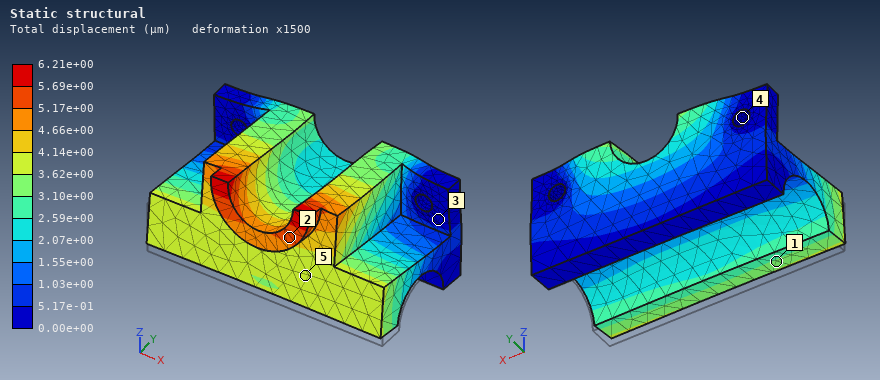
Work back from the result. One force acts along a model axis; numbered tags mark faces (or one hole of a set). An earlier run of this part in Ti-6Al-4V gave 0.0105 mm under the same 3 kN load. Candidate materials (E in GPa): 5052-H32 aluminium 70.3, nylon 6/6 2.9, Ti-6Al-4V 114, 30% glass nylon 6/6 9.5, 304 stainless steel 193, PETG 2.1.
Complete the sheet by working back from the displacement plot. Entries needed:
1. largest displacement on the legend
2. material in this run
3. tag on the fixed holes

6.21e+00 µm
304 stainless steel
4
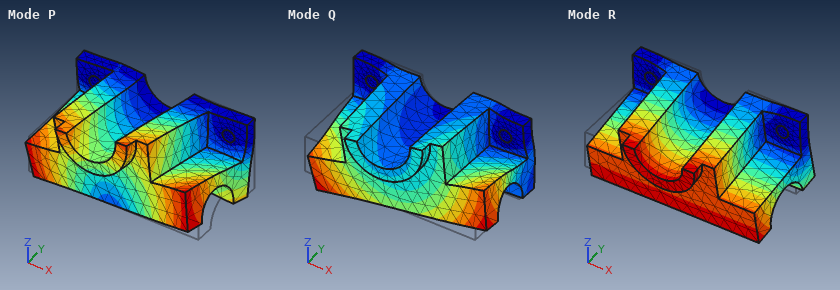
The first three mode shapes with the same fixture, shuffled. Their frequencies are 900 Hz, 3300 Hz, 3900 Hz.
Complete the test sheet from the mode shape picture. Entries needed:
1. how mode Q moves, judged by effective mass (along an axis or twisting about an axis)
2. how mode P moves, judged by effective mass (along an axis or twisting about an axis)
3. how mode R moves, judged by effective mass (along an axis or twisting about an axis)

along X
along X
along Z
